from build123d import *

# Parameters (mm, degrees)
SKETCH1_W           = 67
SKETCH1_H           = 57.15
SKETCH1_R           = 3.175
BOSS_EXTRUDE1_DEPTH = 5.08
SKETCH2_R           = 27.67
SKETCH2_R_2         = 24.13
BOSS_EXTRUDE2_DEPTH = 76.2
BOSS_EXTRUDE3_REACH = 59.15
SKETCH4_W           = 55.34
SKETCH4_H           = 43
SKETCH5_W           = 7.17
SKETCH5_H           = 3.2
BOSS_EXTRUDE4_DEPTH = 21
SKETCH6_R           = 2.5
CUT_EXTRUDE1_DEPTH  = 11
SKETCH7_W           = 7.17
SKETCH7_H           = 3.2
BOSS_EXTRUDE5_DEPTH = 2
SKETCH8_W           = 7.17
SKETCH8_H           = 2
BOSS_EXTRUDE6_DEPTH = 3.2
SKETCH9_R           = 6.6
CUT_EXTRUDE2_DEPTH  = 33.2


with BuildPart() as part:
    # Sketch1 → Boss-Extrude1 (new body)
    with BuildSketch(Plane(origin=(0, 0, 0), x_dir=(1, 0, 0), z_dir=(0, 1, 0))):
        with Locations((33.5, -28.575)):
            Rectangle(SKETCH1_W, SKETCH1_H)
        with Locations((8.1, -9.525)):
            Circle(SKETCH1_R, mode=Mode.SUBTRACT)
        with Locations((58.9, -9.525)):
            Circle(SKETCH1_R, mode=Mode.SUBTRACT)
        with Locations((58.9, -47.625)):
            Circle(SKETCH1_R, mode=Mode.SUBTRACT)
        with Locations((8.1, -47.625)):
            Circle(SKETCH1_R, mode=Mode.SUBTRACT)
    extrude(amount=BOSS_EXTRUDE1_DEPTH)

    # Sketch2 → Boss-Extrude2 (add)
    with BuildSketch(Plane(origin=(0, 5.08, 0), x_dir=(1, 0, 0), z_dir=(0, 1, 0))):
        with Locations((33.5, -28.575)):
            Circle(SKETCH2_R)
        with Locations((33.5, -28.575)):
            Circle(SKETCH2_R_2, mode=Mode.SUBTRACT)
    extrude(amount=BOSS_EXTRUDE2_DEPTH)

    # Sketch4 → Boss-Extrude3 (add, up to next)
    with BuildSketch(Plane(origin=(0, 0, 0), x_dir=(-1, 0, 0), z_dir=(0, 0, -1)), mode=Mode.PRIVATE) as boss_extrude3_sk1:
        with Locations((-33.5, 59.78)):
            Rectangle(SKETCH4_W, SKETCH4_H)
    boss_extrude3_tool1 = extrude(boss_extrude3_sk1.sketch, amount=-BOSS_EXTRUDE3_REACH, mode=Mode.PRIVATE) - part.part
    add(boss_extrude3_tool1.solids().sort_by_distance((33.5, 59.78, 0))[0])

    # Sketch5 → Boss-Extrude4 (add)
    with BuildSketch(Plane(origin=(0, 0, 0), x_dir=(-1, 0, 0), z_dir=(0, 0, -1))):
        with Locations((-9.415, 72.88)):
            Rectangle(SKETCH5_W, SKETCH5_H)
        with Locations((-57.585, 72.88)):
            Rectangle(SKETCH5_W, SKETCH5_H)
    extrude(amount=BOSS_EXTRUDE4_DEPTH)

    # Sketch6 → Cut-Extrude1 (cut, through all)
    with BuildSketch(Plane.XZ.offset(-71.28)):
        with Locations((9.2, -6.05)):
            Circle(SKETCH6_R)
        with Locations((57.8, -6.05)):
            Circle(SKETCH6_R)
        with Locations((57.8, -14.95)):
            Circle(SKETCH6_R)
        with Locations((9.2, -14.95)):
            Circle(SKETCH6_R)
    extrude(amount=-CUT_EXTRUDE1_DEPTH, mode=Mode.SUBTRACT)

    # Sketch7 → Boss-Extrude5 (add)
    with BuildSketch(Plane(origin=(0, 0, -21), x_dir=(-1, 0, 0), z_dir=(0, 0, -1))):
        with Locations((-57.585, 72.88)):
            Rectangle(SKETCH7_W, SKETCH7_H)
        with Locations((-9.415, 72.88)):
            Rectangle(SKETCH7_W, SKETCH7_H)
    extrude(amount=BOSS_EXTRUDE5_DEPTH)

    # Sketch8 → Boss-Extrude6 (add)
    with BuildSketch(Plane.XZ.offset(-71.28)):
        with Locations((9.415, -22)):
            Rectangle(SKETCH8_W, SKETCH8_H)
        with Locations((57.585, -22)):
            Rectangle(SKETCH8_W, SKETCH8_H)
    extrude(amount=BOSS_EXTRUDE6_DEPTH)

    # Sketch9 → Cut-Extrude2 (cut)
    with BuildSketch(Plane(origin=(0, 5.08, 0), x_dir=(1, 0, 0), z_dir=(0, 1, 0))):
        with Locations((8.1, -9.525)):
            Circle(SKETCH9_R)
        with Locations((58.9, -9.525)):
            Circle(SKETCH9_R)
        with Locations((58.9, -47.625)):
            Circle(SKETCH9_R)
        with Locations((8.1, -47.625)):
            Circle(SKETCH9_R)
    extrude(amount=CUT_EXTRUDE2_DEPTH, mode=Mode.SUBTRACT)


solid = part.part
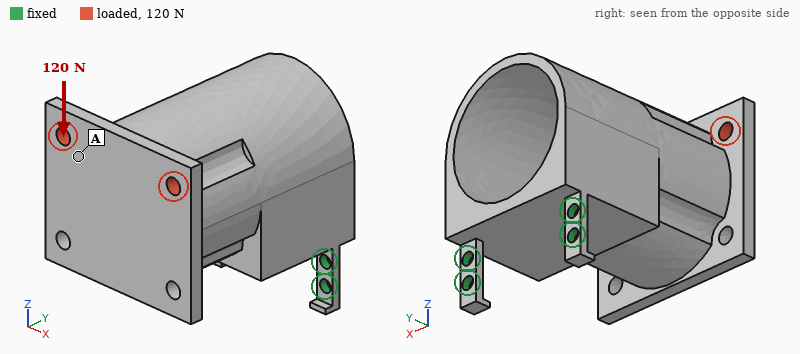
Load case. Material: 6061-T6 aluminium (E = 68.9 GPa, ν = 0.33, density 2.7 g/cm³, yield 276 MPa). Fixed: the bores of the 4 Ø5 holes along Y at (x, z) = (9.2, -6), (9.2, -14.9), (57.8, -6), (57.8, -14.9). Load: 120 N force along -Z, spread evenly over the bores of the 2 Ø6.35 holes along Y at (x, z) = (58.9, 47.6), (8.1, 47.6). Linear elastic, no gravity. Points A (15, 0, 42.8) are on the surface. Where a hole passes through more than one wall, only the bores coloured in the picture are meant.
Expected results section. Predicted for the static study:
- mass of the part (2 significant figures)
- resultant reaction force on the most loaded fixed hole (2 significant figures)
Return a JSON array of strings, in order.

["210 g", "62 N"]
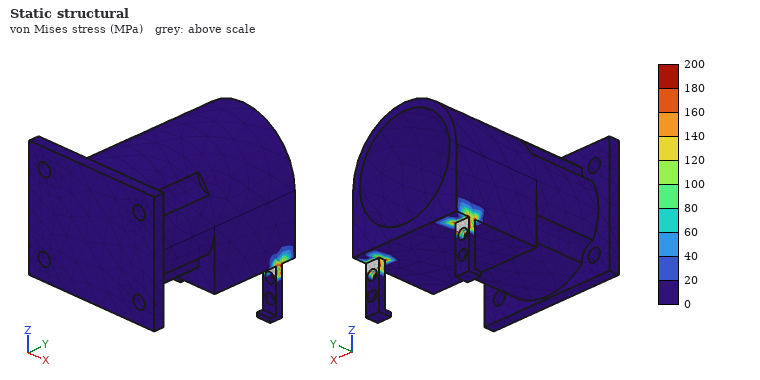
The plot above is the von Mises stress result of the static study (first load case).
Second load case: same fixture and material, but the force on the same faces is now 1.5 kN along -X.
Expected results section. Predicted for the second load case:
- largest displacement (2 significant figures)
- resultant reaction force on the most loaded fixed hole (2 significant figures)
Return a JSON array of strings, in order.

["0.24 mm", "2.7 kN"]
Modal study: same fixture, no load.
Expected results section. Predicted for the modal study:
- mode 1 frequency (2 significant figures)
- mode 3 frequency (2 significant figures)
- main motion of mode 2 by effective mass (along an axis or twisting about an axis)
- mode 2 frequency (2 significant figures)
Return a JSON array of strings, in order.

["150 Hz", "2200 Hz", "along X", "1400 Hz"]
